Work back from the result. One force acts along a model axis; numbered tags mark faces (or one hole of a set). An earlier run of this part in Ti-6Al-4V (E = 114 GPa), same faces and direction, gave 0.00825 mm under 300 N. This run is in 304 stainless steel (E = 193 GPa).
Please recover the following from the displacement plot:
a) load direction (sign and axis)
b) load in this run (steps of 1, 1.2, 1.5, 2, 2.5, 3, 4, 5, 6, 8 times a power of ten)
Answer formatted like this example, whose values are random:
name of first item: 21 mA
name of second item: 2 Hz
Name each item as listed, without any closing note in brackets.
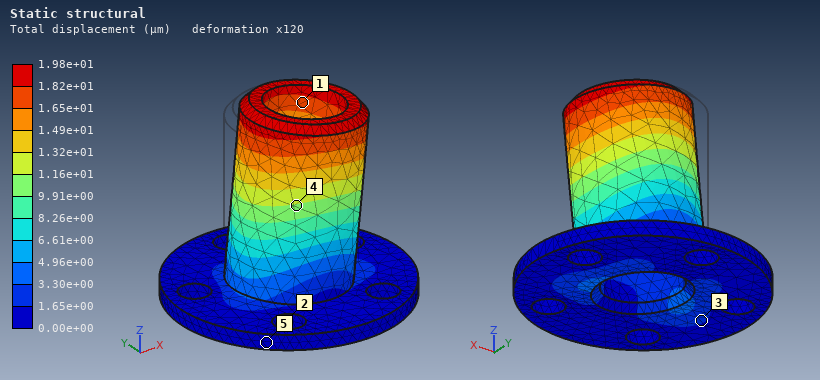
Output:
load direction: +X
load in this run: 1.2 kN
